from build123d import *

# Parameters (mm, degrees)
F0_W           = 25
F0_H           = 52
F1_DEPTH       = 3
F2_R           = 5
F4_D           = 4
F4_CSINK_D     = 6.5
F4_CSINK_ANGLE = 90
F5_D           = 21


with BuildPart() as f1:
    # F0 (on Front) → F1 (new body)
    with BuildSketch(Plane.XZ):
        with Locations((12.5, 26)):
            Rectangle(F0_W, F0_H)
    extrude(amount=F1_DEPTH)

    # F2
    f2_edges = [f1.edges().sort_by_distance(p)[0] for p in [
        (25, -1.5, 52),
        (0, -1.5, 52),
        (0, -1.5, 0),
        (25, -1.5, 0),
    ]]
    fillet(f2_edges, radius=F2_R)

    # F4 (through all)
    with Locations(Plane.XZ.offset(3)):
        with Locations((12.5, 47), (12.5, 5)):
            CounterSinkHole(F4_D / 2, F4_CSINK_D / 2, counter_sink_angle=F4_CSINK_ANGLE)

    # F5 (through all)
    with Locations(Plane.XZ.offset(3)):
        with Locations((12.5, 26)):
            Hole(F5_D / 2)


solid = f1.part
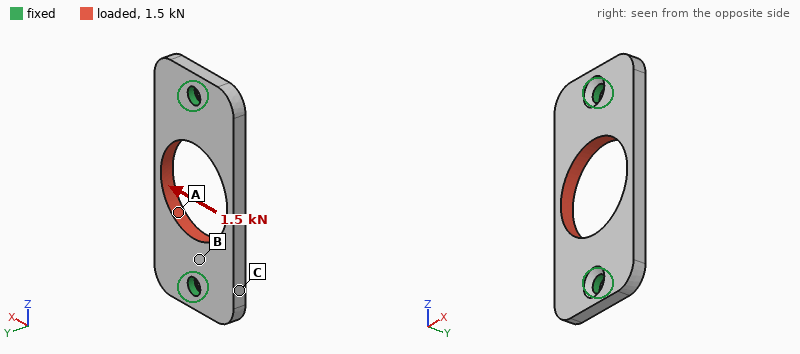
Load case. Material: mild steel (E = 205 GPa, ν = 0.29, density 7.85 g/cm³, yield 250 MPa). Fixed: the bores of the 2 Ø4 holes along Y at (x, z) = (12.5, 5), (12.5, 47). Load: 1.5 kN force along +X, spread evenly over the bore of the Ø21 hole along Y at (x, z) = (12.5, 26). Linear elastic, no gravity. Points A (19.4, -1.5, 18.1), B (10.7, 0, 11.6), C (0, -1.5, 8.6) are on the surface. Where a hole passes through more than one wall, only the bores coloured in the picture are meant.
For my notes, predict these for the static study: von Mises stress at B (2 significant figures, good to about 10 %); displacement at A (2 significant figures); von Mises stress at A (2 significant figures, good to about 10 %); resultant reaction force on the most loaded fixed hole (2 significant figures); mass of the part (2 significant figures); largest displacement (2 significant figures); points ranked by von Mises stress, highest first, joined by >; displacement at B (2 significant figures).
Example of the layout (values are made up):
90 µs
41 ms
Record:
26 MPa
4.9 µm
43 MPa
750 N
21 g
8.2 µm
A > B > C
2.1 µm
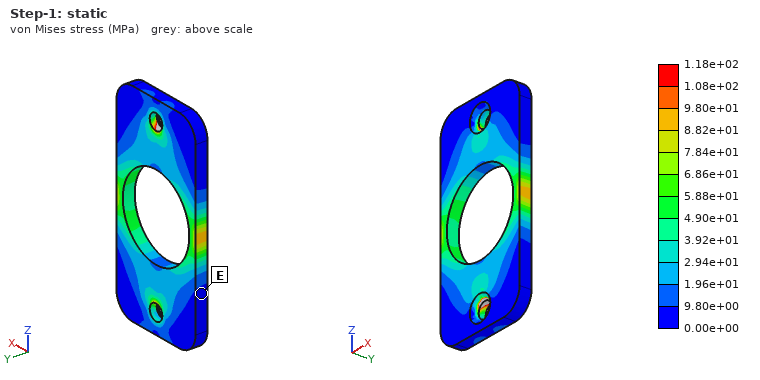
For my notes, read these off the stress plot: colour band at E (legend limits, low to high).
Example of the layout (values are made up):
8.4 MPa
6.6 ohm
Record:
0.00e+00 to 9.80e+00 MPa
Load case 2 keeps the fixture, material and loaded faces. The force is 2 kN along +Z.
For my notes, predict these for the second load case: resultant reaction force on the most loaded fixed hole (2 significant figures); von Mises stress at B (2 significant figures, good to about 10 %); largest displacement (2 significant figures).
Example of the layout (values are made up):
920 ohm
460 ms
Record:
1.0 kN
26 MPa
3.4 µm
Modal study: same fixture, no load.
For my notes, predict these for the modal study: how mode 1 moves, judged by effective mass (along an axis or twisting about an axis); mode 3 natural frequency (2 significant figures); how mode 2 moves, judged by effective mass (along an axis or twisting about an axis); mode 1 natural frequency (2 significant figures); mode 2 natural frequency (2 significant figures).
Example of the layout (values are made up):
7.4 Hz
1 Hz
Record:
twisting about Z
12 kHz
along Y
7600 Hz
8200 Hz
